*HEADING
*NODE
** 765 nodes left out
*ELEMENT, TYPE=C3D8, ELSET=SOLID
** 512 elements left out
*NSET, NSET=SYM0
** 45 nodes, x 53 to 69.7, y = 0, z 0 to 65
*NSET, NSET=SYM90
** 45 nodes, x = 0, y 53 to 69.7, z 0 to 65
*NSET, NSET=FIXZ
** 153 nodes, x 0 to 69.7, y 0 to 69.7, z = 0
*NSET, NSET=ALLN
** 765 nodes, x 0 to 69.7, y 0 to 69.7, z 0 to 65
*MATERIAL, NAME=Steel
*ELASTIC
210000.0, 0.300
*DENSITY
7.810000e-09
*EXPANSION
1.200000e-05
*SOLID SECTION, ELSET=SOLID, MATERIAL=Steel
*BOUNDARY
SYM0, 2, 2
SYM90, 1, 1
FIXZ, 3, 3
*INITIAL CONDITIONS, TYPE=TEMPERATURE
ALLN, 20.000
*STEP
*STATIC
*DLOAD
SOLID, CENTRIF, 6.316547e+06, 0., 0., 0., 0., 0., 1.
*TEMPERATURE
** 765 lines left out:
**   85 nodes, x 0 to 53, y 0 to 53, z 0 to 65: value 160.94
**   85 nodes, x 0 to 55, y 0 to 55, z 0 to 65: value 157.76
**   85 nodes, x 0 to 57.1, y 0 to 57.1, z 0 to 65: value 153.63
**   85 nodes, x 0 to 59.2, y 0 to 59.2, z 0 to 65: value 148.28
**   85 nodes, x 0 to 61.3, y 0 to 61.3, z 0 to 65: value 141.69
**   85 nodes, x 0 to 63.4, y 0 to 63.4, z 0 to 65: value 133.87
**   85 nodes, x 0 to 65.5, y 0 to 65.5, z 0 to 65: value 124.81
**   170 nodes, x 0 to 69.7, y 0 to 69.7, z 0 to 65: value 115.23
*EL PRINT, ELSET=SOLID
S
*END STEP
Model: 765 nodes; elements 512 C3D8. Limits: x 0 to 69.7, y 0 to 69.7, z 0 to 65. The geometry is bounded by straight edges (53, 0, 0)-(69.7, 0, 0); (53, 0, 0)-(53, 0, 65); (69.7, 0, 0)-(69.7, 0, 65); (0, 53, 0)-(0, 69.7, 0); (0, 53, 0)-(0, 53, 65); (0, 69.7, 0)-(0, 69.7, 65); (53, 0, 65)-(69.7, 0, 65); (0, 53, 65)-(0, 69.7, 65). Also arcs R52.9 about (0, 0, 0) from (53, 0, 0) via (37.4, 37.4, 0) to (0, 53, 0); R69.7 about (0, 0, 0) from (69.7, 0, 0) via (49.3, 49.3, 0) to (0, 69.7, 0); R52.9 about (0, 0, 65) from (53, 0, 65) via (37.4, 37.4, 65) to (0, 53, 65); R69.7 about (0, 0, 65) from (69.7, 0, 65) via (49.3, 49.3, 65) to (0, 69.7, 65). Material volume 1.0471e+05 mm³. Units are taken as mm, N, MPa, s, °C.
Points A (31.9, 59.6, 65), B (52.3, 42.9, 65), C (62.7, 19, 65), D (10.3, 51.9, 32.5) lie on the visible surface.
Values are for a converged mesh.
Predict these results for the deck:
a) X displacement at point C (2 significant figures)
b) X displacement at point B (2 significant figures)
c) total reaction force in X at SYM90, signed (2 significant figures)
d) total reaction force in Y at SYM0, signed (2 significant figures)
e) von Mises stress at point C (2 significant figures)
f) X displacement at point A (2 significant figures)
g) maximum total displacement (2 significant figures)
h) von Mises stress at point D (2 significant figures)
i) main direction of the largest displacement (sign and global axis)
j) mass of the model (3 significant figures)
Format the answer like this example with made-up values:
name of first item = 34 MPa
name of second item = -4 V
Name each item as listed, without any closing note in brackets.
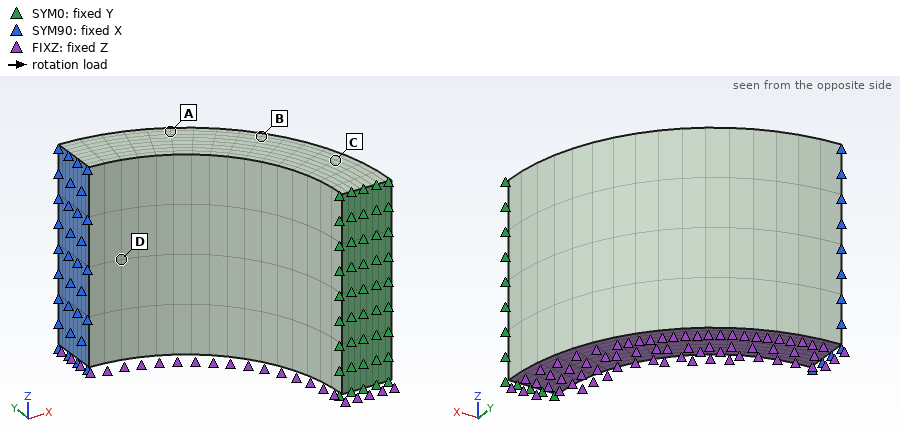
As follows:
X displacement at point C = 0.15 mm
X displacement at point B = 0.13 mm
total reaction force in X at SYM90, signed = -2.0e+05 N
total reaction force in Y at SYM0, signed = -2.0e+05 N
von Mises stress at point C = 250 MPa
X displacement at point A = 0.076 mm
maximum total displacement = 0.18 mm
von Mises stress at point D = 170 MPa
main direction of the largest displacement = +X
mass of the model = 0.818 kg
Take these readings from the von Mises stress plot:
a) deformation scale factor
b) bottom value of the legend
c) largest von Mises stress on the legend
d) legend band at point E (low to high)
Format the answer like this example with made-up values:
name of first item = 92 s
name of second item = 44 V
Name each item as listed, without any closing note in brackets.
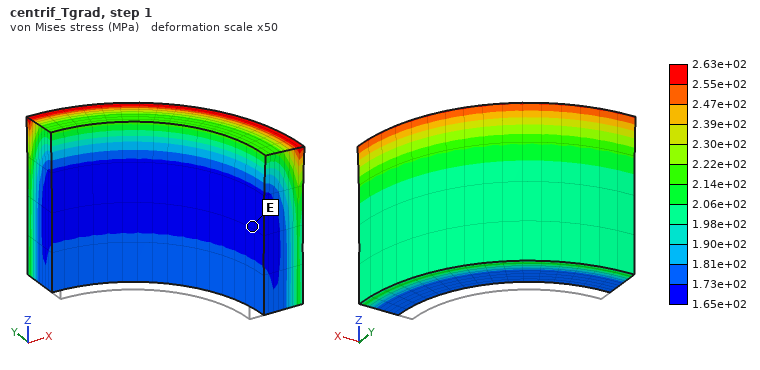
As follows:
deformation scale factor = 50
bottom value of the legend = 1.65e+02 MPa
largest von Mises stress on the legend = 2.63e+02 MPa
legend band at point E = 1.65e+02 to 1.73e+02 MPa
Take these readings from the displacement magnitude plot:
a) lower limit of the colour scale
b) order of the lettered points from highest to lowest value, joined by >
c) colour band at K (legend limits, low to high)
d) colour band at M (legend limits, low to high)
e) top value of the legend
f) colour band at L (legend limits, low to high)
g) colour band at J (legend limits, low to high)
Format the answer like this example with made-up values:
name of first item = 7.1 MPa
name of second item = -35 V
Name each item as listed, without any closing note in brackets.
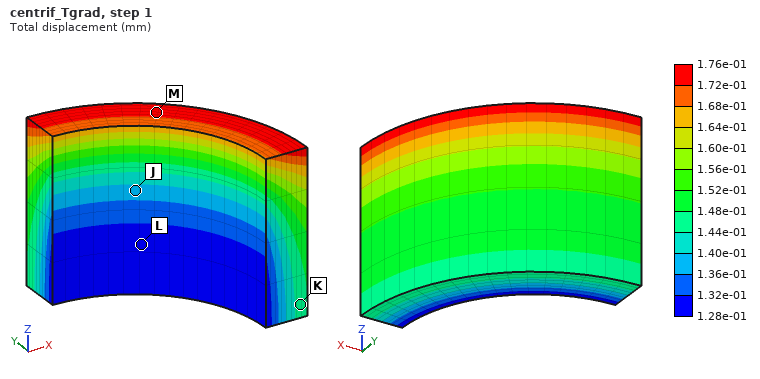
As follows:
lower limit of the colour scale = 1.28e-01 mm
order of the lettered points from highest to lowest value, joined by > = M > K > J > L
colour band at K = 1.44e-01 to 1.48e-01 mm
colour band at M = 1.72e-01 to 1.76e-01 mm
top value of the legend = 1.76e-01 mm
colour band at L = 1.28e-01 to 1.32e-01 mm
colour band at J = 1.36e-01 to 1.40e-01 mm
